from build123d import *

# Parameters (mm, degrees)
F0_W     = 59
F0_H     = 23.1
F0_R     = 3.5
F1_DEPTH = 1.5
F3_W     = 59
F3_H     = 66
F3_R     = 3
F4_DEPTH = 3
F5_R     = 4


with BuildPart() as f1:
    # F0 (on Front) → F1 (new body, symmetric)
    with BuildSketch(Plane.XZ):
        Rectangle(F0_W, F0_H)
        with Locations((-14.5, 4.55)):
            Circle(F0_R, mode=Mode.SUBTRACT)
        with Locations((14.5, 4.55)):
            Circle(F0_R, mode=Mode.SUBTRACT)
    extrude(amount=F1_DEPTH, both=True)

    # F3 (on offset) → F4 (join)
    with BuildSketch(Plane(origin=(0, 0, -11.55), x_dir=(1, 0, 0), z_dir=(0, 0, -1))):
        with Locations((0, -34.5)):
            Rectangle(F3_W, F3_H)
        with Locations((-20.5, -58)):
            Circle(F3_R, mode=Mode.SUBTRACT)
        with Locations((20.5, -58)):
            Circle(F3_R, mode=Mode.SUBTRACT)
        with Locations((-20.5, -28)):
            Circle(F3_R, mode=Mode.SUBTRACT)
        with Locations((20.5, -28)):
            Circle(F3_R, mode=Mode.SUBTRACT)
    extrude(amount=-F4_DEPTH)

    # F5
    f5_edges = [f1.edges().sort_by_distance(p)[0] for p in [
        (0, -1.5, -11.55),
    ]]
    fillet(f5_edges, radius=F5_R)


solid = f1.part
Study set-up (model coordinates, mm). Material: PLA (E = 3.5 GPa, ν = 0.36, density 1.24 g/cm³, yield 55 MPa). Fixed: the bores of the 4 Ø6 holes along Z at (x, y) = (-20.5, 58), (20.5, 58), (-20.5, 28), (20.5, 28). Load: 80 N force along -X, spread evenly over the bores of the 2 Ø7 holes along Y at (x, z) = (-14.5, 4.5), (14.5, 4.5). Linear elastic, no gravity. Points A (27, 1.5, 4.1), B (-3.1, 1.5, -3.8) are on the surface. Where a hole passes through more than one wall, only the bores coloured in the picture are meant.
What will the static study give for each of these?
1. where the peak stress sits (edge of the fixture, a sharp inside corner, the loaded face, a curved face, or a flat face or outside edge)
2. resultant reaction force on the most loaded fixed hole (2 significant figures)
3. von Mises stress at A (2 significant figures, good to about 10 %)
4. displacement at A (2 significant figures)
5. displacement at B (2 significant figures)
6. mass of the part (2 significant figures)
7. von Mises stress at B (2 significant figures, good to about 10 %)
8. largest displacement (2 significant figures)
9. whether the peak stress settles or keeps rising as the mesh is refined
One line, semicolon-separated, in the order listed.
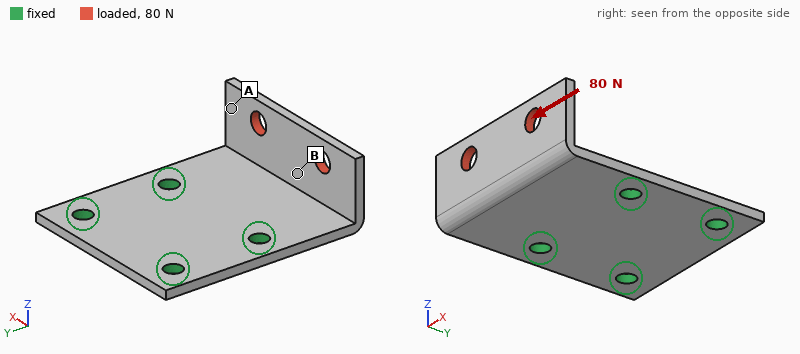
edge of the fixture; 66 N; 2.1 MPa; 0.55 mm; 0.14 mm; 19 g; 4.7 MPa; 0.70 mm; keeps rising
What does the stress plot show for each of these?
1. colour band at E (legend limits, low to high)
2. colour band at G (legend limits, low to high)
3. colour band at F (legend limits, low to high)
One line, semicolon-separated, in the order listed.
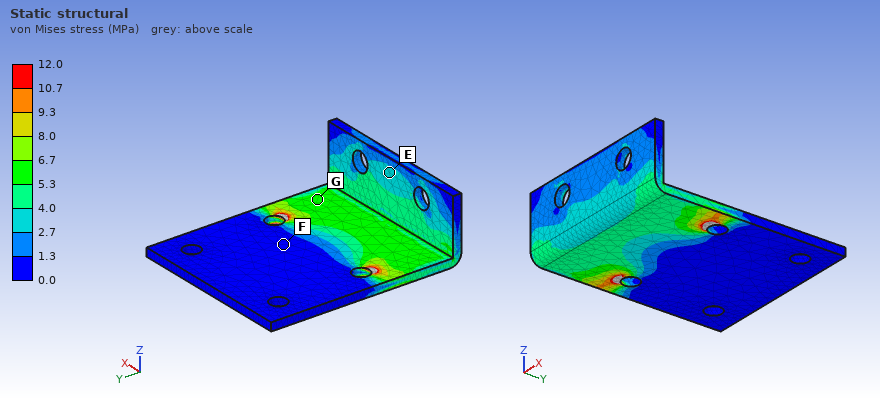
2.7 to 4.0 MPa; 5.3 to 6.7 MPa; 0.0 to 1.3 MPa
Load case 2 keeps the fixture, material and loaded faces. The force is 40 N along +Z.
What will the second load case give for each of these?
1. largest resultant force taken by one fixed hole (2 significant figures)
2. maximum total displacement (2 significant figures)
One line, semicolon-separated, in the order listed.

23 N; 0.91 mm
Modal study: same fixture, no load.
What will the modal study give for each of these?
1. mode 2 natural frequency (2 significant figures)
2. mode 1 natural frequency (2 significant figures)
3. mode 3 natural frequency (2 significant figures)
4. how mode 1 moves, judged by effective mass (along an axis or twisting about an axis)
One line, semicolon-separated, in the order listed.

810 Hz; 470 Hz; 1400 Hz; along Z
